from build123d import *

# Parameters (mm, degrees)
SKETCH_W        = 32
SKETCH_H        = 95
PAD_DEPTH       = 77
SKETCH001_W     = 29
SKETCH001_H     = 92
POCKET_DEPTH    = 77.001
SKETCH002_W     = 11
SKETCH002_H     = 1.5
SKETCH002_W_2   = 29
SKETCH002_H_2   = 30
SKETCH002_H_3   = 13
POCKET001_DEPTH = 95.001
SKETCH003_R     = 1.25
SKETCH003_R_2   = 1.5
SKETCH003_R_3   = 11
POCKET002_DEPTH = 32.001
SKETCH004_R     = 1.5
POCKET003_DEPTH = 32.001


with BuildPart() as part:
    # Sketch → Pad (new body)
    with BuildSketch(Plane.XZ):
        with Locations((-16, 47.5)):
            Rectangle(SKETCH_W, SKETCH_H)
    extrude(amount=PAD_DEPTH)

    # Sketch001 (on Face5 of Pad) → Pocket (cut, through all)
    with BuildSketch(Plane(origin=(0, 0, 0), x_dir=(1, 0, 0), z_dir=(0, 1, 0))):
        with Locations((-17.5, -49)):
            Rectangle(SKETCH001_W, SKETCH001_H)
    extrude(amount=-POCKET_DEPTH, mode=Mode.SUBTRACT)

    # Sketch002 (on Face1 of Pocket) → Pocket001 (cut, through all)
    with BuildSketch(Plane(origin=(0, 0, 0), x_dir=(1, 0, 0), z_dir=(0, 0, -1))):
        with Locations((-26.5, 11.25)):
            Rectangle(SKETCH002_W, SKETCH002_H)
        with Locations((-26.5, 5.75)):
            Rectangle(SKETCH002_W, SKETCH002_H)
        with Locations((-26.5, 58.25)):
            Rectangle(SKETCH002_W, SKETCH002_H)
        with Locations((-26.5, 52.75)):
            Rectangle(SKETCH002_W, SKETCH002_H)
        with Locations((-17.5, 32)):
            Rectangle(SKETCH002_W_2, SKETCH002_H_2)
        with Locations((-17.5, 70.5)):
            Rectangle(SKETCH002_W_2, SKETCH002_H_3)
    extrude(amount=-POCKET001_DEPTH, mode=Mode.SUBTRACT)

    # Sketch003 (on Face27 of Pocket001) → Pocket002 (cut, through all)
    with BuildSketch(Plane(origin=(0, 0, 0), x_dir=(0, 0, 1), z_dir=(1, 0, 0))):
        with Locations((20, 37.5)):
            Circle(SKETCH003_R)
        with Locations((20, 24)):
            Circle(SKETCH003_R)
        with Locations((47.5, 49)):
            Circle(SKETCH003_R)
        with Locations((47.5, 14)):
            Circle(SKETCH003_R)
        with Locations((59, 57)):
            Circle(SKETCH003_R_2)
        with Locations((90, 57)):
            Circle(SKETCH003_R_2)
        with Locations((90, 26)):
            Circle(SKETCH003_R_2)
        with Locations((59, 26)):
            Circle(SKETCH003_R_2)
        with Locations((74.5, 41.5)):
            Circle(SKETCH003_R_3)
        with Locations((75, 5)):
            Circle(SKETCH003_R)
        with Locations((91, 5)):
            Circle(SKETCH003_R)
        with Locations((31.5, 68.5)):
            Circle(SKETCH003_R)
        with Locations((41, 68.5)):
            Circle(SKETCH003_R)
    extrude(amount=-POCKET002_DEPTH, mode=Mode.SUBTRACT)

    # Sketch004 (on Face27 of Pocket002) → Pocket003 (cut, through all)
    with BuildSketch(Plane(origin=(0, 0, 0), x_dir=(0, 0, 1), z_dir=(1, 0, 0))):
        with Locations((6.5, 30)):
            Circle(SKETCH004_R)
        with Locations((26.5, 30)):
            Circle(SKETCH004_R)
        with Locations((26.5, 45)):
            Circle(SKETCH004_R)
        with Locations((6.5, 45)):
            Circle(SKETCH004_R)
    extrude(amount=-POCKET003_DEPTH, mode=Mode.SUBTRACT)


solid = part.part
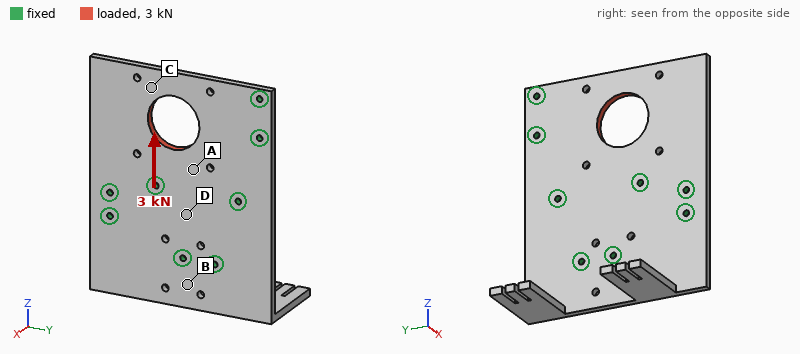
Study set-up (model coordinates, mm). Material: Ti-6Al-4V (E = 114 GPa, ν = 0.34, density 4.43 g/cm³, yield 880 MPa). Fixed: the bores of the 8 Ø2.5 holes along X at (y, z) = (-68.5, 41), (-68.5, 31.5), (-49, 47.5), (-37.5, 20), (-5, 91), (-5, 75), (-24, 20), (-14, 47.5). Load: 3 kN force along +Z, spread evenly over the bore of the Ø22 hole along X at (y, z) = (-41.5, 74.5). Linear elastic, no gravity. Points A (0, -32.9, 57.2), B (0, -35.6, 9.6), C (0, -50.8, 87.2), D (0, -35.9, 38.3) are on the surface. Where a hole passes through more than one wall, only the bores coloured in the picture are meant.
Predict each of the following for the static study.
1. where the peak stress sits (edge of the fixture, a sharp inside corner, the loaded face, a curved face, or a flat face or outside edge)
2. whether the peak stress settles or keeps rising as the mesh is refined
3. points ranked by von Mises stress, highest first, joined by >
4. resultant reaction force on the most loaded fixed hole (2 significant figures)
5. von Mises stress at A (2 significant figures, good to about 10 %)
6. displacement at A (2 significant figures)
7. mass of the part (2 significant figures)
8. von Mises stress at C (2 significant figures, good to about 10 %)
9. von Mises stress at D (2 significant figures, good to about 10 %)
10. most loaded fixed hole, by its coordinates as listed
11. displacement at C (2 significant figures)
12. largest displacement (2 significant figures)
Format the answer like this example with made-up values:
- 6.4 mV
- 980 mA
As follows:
- edge of the fixture
- keeps rising
- C > A > D > B
- 850 N
- 14 MPa
- 2.7 µm
- 100 g
- 20 MPa
- 7.2 MPa
- (-49, 47.5)
- 9.3 µm
- 12 µm
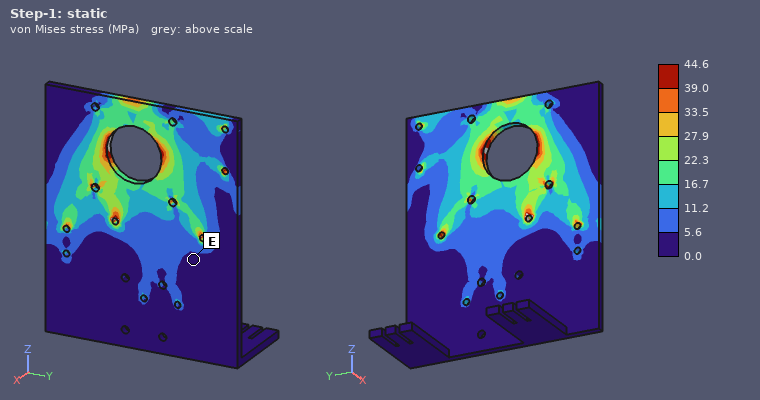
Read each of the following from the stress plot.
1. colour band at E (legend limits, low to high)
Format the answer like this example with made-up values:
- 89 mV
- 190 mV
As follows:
- 0.0 to 5.6 MPa
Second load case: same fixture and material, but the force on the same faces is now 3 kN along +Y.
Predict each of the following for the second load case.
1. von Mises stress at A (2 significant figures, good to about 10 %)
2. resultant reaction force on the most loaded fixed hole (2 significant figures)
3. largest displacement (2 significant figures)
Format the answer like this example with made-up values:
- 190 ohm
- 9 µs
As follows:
- 16 MPa
- 810 N
- 11 µm
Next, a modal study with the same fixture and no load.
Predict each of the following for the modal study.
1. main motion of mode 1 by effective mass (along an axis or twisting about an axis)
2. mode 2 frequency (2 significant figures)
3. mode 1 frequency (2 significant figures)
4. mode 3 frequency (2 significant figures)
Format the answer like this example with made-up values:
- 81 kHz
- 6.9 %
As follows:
- along X
- 1500 Hz
- 1300 Hz
- 1700 Hz
